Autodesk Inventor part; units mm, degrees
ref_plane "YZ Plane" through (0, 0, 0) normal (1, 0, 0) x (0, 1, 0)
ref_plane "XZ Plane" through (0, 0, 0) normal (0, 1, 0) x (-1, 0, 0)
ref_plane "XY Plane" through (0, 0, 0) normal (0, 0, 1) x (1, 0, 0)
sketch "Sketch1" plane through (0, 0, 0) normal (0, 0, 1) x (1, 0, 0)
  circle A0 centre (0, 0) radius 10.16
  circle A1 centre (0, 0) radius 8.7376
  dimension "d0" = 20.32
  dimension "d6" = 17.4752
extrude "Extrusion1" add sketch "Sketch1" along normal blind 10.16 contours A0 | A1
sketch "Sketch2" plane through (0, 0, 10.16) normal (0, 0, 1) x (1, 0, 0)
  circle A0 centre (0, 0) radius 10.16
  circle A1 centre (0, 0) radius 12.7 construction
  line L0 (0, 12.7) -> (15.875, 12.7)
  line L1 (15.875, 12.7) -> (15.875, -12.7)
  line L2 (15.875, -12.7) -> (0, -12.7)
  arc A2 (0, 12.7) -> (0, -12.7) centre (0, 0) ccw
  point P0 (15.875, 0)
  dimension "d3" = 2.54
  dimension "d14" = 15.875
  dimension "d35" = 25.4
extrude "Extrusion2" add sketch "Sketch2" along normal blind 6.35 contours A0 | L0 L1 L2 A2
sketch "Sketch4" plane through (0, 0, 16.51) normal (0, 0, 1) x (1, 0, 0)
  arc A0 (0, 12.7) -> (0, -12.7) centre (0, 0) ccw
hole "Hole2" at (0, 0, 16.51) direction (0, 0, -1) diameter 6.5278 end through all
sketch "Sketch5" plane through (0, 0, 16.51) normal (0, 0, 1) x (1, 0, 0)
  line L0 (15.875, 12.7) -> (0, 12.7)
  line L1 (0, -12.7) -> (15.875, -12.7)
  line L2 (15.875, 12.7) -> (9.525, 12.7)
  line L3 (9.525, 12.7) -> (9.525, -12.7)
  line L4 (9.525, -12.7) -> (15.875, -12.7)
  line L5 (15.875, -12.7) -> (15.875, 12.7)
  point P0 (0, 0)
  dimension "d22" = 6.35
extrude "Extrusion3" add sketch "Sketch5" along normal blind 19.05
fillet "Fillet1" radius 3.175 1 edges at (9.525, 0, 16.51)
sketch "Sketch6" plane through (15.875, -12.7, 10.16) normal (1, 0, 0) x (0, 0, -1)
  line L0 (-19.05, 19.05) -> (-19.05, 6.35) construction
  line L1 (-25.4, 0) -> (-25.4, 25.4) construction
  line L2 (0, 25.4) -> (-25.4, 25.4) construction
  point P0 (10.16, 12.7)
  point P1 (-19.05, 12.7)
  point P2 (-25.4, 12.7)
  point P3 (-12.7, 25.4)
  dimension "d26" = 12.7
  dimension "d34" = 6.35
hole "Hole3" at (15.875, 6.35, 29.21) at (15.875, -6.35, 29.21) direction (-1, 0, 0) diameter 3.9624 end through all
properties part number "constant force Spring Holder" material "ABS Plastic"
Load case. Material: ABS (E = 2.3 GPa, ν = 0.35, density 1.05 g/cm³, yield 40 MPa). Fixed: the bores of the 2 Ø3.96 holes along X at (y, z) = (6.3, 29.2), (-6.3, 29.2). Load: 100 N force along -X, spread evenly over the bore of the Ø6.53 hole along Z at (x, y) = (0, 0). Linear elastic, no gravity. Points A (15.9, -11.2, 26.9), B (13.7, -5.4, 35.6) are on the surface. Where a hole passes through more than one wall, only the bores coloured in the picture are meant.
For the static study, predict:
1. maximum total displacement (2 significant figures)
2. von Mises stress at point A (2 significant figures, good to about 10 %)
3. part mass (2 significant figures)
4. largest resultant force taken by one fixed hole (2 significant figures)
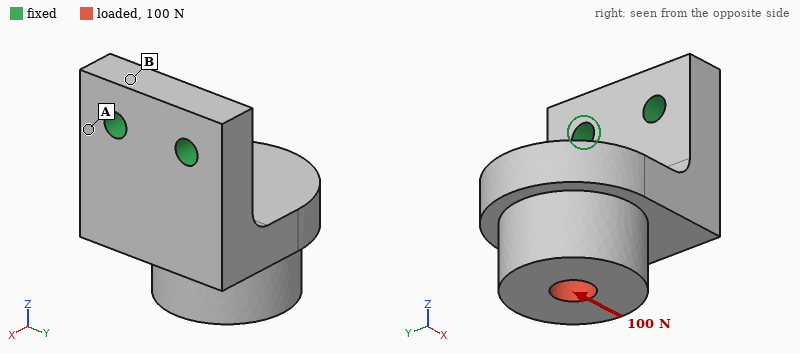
0.53 mm
6.8 MPa
10 g
50 N
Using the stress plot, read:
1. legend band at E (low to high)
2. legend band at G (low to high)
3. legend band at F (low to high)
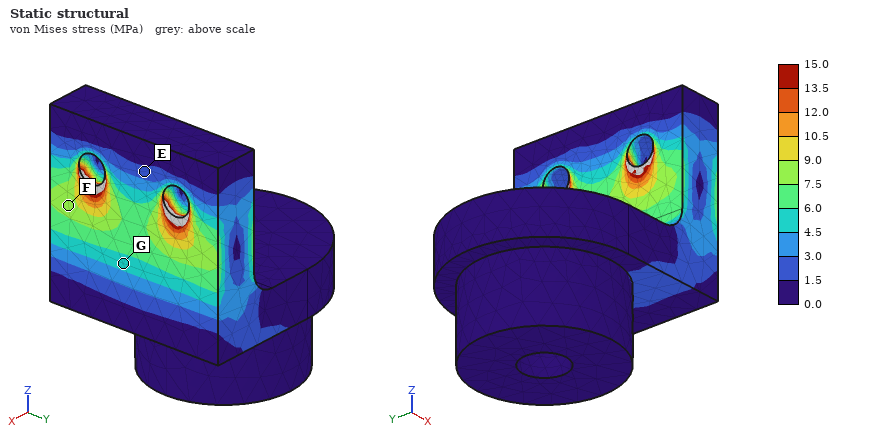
1.5 to 3.0 MPa
4.5 to 6.0 MPa
7.5 to 9.0 MPa
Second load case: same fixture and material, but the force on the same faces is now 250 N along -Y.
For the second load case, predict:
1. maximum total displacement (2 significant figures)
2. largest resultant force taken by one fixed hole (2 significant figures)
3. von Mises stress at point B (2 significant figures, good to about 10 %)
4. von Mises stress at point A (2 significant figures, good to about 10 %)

0.41 mm
390 N
2.7 MPa
11 MPa
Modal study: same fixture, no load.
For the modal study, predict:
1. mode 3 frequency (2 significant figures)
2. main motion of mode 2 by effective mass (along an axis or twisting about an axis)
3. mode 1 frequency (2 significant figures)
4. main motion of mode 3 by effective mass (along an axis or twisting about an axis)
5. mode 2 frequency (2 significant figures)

3800 Hz
along Y
920 Hz
along X
1800 Hz
